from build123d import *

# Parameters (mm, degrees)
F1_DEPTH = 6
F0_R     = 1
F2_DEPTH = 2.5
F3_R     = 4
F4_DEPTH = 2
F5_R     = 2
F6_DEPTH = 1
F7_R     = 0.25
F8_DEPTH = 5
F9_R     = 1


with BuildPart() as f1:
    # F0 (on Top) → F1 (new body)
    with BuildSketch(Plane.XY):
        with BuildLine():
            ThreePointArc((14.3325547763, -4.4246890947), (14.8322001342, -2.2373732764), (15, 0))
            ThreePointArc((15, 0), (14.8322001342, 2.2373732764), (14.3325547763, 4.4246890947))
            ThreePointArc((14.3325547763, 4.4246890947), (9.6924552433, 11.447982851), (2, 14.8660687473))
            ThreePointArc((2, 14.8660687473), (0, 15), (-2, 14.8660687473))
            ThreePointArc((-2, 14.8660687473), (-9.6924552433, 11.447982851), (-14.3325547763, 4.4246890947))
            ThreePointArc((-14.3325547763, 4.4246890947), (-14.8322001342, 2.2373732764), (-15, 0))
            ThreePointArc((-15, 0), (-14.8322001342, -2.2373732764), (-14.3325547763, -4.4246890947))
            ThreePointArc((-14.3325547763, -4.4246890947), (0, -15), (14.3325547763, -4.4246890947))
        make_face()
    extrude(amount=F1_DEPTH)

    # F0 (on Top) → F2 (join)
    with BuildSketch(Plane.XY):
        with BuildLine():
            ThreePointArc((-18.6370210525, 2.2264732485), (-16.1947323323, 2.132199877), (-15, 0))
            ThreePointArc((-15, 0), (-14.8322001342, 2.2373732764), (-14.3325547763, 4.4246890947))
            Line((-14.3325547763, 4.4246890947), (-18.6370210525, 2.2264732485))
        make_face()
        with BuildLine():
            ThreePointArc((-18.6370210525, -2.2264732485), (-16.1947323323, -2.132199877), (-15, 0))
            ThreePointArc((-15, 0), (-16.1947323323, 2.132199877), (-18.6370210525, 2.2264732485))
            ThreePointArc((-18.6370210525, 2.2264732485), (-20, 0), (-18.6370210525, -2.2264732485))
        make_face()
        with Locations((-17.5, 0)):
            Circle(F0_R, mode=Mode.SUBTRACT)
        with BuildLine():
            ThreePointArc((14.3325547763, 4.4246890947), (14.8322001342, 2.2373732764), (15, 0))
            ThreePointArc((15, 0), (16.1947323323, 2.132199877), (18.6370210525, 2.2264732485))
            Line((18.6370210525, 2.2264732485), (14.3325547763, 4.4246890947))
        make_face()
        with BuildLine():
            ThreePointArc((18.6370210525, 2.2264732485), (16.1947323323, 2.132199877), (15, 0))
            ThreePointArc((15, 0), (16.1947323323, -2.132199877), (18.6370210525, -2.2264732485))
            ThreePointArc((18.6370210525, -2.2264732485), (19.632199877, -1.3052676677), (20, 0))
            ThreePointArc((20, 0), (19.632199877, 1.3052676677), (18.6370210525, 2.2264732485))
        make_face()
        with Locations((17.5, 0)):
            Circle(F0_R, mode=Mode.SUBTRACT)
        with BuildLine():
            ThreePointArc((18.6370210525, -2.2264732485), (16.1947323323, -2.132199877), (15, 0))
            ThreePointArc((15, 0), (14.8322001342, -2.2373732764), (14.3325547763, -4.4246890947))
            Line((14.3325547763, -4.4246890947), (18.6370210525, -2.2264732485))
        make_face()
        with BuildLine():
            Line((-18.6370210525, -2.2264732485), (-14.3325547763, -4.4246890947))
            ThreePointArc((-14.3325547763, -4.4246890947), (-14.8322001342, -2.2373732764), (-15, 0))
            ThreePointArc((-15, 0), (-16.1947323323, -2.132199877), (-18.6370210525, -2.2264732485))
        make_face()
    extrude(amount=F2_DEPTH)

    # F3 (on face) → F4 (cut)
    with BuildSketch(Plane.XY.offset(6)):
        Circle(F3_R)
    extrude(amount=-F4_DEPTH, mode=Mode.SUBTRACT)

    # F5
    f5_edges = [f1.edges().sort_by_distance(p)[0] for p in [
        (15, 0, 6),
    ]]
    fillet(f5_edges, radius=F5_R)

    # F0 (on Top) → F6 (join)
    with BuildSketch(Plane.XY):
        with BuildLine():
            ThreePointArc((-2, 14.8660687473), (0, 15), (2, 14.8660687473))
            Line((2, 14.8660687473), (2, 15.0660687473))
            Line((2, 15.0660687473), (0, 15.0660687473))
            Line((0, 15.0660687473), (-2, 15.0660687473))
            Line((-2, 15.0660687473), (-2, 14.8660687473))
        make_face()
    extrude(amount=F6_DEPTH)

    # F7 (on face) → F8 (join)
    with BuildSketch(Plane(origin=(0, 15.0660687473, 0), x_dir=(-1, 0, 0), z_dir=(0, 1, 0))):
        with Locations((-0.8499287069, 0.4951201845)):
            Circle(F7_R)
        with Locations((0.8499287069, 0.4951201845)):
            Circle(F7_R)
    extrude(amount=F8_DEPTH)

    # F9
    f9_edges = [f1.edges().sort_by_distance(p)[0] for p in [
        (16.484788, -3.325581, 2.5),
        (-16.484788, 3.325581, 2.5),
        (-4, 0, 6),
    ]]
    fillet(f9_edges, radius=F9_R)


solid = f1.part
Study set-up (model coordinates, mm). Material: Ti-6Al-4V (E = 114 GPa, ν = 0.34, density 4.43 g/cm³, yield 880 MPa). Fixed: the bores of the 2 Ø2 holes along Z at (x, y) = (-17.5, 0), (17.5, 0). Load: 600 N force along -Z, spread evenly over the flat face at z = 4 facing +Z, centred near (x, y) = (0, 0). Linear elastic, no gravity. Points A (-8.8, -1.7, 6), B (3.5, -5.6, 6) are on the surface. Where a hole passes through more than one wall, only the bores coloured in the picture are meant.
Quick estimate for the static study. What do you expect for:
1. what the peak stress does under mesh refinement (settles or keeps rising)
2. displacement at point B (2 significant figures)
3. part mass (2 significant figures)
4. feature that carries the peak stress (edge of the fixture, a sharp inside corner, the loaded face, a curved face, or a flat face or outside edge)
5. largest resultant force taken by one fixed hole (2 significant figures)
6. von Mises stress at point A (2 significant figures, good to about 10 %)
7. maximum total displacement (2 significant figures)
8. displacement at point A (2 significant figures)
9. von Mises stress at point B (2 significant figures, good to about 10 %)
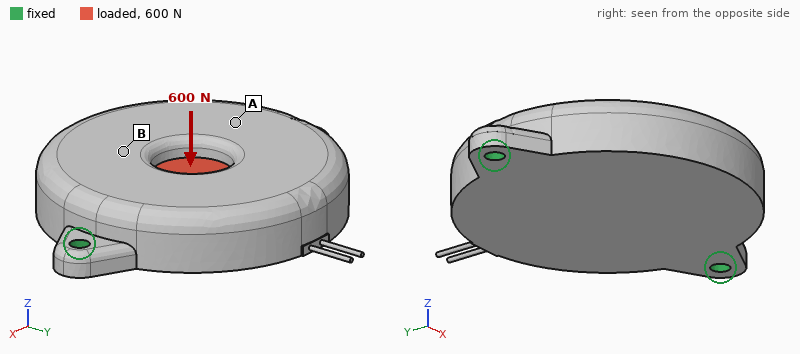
keeps rising
9.9 µm
19 g
edge of the fixture
430 N
15 MPa
12 µm
7.6 µm
28 MPa
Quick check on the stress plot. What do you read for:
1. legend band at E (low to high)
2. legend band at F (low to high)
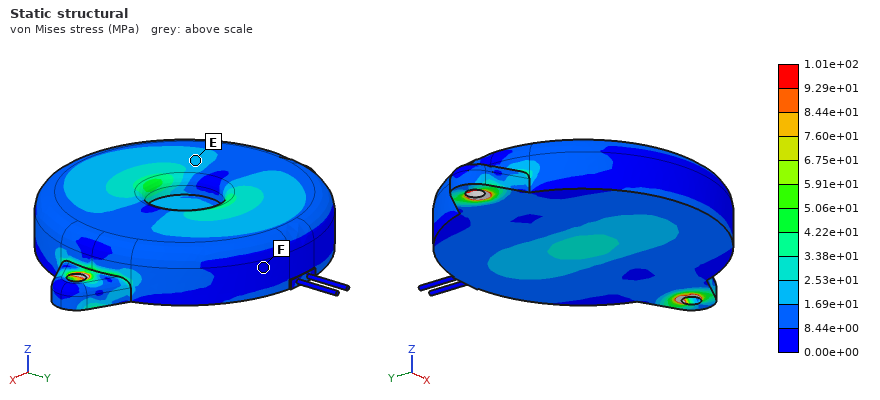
1.69e+01 to 2.53e+01 MPa
0.00e+00 to 8.44e+00 MPa
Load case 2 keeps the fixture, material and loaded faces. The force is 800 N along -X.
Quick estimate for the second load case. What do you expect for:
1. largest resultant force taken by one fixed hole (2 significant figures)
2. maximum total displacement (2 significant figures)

410 N
2.5 µm
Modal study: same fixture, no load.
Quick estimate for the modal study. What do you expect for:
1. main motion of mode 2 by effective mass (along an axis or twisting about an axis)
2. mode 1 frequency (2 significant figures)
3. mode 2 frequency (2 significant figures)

along Z
4400 Hz
10 kHz
